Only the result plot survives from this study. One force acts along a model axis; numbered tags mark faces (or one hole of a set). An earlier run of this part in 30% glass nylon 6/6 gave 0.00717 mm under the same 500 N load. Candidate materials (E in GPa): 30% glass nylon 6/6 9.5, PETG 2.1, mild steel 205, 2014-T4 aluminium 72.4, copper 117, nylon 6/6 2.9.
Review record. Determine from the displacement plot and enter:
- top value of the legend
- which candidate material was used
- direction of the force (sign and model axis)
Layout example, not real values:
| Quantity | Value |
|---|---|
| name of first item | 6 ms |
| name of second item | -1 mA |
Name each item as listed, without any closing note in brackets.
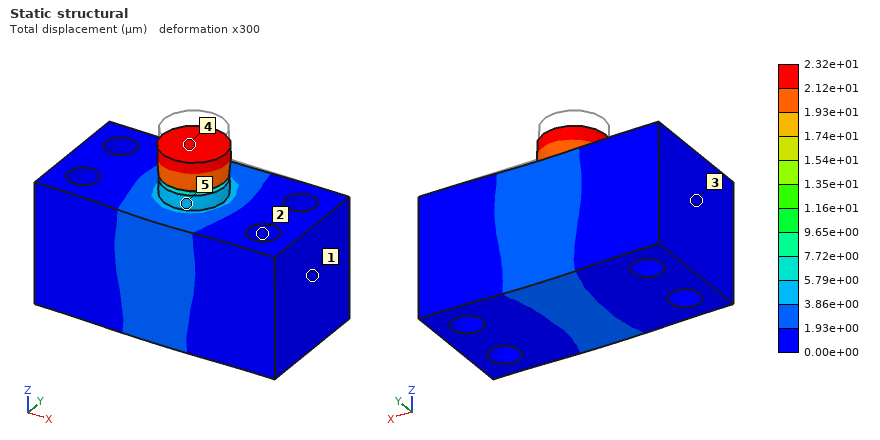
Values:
| Quantity | Value |
|---|---|
| top value of the legend | 2.32e+01 µm |
| which candidate material was used | nylon 6/6 |
| direction of the force | -Z |
